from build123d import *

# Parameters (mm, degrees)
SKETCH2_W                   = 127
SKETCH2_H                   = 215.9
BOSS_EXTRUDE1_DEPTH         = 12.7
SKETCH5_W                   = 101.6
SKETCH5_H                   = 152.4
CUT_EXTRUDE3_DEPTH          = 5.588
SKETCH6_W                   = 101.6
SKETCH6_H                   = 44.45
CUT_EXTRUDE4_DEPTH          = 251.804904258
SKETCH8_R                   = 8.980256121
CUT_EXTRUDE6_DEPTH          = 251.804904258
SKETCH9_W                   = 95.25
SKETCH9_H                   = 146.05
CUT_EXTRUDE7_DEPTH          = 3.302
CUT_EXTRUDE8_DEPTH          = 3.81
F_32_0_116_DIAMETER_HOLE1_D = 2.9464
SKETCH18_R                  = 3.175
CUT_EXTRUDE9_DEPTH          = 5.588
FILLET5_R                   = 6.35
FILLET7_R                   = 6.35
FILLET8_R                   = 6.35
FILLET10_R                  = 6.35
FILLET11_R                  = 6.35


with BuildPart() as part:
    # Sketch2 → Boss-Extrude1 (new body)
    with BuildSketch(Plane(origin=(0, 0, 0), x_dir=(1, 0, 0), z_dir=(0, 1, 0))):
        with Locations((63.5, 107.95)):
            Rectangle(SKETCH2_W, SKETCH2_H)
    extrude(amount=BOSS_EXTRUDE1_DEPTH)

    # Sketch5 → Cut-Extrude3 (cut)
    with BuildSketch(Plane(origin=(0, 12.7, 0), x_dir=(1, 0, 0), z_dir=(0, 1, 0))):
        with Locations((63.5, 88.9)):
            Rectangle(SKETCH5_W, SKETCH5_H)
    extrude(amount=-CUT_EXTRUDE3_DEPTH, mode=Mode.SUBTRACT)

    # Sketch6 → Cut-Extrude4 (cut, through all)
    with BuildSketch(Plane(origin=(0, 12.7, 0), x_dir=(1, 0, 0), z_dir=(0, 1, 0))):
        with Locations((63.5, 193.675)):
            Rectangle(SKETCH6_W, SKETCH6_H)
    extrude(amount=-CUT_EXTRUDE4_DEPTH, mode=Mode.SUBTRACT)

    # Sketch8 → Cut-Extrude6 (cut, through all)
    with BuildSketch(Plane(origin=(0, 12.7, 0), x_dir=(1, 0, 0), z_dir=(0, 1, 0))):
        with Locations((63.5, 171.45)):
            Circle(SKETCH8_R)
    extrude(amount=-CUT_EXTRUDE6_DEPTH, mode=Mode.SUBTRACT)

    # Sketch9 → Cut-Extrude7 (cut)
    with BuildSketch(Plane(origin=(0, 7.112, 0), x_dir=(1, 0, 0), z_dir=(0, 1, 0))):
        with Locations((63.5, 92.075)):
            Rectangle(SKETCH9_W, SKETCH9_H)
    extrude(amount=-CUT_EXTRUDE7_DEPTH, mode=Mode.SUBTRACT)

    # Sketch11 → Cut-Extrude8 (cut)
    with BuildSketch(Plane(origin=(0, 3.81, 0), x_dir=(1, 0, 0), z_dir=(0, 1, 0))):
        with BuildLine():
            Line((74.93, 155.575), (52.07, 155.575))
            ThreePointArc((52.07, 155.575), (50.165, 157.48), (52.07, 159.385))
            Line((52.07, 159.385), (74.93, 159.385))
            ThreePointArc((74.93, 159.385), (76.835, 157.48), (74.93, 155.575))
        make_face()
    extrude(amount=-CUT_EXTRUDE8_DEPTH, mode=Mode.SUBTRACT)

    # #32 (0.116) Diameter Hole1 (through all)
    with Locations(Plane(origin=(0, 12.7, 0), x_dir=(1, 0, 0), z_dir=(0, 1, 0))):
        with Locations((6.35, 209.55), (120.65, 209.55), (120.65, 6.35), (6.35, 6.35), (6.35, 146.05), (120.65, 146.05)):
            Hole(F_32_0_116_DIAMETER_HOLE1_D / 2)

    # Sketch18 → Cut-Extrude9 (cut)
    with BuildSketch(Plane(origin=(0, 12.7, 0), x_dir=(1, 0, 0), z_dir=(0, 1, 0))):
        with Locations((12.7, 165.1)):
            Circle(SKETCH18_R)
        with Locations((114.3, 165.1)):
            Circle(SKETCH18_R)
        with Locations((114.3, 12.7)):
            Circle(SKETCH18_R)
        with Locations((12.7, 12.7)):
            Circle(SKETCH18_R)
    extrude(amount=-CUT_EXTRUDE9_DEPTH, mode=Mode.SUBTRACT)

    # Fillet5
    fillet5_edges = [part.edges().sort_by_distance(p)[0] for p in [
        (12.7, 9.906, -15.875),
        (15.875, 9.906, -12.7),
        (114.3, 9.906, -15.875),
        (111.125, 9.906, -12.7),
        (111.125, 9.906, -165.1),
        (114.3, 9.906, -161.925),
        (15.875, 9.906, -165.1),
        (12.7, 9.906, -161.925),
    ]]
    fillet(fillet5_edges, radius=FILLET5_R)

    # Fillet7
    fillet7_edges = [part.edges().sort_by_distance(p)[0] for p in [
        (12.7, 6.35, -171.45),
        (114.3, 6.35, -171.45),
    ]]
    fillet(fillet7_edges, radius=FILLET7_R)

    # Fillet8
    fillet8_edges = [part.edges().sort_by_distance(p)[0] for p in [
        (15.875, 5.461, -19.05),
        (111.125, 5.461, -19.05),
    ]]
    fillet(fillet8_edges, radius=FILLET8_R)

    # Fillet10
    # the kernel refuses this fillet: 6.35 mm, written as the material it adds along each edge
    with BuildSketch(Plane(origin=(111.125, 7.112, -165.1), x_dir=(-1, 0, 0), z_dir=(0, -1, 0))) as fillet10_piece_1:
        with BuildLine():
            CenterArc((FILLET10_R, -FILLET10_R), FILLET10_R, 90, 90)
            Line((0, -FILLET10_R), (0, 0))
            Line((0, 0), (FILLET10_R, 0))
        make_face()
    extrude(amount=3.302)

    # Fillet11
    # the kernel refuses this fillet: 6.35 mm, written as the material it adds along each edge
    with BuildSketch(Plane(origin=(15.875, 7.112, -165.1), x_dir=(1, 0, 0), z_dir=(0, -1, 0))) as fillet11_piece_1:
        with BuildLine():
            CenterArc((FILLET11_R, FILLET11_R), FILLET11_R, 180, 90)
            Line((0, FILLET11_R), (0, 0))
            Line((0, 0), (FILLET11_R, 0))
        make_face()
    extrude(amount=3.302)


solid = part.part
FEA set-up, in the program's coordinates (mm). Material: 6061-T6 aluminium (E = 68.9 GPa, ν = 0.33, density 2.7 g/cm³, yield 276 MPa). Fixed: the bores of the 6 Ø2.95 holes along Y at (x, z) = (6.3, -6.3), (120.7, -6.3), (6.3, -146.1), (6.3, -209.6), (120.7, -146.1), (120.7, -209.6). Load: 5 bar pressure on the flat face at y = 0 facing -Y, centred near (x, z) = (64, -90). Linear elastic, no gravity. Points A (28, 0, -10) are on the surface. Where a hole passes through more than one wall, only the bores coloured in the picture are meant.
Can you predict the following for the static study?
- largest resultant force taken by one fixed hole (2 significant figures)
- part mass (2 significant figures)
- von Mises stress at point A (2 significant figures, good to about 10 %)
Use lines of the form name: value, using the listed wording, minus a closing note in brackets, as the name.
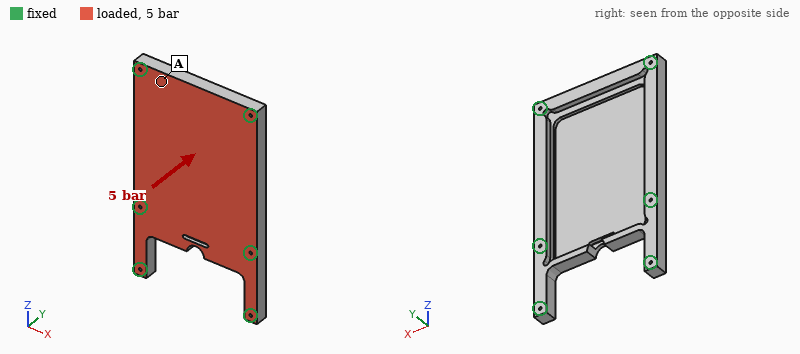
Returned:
largest resultant force taken by one fixed hole: 4.4 kN
part mass: 420 g
von Mises stress at point A: 21 MPa
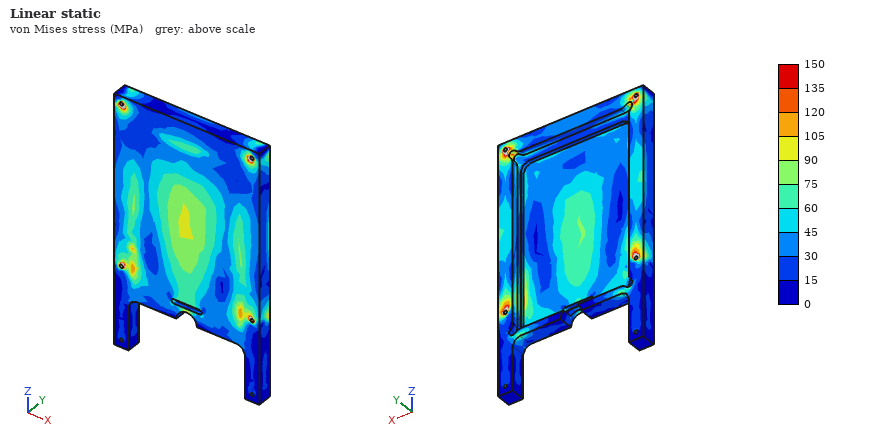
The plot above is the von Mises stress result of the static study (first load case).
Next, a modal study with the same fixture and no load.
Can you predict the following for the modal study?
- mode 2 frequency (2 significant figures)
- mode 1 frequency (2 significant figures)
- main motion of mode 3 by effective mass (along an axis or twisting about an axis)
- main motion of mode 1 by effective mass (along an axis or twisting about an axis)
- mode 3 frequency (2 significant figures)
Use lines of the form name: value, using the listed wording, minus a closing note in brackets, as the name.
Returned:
mode 2 frequency: 2600 Hz
mode 1 frequency: 1700 Hz
main motion of mode 3 by effective mass: twisting about Z
main motion of mode 1 by effective mass: along Y
mode 3 frequency: 2700 Hz
